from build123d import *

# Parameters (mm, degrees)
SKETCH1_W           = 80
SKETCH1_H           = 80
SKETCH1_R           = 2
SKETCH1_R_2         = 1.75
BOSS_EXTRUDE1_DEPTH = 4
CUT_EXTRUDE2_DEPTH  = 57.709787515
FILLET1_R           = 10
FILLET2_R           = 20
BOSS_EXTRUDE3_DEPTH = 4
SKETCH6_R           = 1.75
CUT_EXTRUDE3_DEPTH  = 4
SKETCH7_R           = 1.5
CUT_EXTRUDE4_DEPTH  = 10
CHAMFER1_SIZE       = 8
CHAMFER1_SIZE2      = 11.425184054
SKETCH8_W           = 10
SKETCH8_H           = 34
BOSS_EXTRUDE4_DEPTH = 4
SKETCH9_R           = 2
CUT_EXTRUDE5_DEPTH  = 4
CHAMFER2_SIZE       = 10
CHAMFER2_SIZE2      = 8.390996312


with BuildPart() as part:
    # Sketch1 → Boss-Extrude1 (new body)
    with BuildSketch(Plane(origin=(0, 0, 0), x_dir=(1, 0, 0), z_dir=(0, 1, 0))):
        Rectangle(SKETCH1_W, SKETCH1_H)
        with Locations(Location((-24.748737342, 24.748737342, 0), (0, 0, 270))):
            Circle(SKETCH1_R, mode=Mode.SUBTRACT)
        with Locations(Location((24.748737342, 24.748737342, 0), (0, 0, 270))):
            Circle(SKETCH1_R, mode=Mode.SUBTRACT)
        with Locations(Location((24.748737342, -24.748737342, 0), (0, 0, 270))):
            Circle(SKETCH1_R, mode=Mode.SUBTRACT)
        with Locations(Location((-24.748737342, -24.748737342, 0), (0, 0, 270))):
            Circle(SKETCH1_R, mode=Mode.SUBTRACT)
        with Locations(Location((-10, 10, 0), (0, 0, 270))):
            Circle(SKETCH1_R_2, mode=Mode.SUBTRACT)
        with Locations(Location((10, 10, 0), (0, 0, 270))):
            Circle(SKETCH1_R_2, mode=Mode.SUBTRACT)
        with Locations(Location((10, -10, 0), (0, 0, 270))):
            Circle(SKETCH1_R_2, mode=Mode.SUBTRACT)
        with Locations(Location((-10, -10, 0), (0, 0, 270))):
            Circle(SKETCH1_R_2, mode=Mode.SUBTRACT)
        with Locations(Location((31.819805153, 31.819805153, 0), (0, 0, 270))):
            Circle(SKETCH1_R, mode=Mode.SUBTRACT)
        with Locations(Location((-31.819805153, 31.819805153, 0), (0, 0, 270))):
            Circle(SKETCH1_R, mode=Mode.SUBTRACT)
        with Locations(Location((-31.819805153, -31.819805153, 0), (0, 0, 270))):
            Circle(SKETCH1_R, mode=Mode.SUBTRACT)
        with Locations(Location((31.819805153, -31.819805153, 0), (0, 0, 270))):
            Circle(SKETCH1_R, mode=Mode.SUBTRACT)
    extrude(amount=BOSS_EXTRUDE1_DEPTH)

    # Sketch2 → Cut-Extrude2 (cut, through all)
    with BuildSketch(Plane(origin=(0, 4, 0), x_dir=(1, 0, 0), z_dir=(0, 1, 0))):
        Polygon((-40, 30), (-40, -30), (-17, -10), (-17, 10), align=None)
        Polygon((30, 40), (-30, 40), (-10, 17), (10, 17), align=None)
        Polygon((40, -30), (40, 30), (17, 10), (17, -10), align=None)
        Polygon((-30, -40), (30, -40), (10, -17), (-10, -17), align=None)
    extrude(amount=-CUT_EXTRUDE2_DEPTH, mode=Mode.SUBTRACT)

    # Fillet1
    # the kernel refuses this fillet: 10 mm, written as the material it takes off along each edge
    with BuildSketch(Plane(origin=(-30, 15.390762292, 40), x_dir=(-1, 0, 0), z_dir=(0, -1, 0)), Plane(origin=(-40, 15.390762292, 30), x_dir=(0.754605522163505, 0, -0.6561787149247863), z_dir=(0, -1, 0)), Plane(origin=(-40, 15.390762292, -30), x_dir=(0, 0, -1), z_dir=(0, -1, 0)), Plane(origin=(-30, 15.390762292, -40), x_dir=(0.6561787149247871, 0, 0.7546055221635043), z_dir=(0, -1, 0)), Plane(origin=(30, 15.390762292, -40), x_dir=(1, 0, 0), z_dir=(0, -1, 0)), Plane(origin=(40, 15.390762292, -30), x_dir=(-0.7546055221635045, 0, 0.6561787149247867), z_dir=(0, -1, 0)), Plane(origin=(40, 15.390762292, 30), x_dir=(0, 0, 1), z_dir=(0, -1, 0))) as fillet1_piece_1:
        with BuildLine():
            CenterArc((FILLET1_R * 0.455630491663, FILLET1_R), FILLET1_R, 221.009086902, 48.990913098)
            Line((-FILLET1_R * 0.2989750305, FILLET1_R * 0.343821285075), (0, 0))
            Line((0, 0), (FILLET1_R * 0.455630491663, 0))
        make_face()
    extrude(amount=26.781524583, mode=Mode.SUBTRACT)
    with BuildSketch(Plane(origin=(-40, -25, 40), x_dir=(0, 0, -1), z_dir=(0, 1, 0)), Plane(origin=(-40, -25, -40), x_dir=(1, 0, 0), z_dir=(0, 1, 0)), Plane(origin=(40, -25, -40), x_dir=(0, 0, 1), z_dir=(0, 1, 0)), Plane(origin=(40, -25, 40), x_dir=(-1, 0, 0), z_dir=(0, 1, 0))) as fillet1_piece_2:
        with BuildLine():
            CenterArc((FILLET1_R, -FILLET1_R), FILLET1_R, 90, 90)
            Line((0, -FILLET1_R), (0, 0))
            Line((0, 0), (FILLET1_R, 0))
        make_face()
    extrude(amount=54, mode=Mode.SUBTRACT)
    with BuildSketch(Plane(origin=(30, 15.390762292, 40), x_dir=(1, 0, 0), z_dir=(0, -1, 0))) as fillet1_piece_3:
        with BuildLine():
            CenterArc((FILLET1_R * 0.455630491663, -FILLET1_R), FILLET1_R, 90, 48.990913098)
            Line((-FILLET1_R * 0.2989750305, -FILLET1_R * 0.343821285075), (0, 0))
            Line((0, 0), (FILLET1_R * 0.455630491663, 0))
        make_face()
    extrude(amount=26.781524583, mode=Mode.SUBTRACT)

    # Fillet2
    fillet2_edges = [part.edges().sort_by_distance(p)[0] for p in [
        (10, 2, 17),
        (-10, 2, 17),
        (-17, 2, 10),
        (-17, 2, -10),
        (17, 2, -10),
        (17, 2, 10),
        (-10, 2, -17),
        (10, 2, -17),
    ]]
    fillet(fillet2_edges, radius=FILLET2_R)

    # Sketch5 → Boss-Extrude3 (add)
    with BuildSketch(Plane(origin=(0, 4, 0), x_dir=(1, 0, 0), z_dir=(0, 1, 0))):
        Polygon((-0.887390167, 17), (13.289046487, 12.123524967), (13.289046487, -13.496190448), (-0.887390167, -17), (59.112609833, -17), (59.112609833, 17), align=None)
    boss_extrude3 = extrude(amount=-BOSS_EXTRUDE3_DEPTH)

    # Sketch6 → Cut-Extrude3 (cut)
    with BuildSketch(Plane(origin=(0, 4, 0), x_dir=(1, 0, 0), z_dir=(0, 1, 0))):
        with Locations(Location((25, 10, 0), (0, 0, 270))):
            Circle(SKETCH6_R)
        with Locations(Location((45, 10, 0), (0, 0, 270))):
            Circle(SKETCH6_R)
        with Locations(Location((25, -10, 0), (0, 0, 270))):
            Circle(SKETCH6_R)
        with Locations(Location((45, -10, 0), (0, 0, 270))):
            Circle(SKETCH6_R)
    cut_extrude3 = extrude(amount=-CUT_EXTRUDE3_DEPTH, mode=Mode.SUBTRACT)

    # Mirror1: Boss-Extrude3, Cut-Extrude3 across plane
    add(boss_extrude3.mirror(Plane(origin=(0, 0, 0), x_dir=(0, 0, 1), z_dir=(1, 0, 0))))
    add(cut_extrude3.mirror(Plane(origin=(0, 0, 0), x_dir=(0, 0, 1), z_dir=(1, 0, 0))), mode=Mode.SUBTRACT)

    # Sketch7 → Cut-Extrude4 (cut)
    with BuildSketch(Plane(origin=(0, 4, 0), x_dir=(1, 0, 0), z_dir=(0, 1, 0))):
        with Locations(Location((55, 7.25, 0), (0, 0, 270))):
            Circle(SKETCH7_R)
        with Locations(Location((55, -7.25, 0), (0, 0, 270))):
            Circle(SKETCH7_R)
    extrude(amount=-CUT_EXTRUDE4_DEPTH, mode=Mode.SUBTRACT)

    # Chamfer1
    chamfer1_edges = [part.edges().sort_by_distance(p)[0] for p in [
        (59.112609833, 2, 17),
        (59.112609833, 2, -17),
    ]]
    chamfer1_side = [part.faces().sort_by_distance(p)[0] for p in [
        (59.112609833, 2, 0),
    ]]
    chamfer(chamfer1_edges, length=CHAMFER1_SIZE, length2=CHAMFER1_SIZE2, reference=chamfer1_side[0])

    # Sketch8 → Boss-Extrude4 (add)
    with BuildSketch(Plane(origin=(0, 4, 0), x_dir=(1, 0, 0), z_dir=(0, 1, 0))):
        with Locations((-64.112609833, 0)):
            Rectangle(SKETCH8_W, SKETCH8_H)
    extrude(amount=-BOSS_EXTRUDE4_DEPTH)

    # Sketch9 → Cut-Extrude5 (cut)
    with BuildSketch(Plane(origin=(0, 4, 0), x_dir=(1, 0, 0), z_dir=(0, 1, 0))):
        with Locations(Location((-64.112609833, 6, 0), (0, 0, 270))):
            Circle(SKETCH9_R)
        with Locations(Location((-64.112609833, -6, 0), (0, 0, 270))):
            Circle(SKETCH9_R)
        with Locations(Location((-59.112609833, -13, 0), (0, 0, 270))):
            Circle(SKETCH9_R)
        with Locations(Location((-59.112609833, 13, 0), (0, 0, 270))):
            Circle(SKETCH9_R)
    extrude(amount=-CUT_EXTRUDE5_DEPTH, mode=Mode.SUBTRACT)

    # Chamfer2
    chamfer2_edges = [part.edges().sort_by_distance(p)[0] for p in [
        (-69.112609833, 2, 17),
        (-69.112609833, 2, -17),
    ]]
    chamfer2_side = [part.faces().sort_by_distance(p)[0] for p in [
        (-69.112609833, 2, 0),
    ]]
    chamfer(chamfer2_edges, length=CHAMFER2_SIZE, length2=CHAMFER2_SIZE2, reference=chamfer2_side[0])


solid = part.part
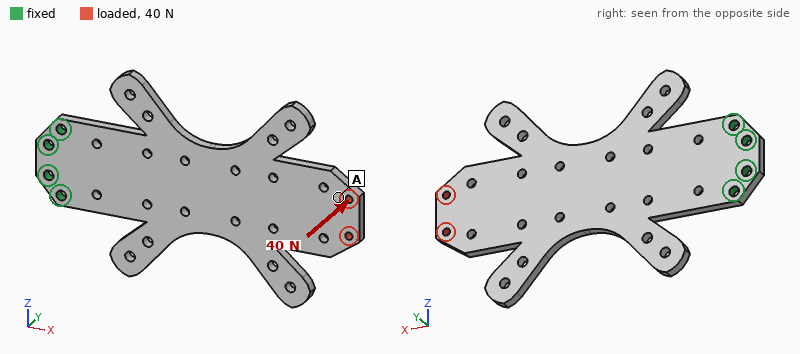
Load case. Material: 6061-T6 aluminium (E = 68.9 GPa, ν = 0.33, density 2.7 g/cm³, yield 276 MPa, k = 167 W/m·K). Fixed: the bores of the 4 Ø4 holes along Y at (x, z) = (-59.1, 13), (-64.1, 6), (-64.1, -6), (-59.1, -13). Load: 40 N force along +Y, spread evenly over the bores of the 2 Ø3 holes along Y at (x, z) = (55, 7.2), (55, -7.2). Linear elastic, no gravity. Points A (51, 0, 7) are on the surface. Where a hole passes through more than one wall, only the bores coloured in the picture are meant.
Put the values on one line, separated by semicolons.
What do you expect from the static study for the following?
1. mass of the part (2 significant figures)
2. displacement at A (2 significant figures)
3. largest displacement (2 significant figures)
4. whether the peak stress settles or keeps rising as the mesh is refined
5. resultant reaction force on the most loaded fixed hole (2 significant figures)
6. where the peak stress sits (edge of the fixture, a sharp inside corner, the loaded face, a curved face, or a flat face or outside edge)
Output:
57 g; 1.5 mm; 1.7 mm; keeps rising; 86 N; edge of the fixture
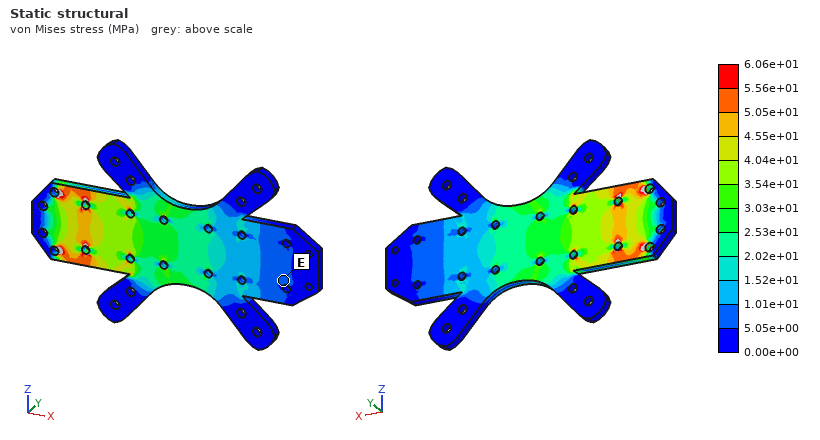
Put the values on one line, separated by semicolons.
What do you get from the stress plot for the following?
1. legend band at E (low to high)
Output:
5.05e+00 to 1.01e+01 MPa
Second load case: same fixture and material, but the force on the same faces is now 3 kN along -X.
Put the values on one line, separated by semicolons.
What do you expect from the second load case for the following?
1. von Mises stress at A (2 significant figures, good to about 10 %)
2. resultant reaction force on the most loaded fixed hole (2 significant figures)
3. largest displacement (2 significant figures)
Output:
38 MPa; 950 N; 43 µm
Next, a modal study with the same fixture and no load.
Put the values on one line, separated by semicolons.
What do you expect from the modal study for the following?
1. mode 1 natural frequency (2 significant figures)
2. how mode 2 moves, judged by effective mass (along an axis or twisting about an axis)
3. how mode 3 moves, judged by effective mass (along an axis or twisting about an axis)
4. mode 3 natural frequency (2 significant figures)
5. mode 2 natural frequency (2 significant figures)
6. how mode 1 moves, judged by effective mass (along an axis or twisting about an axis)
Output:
220 Hz; twisting about X; along Y; 1400 Hz; 850 Hz; along Y
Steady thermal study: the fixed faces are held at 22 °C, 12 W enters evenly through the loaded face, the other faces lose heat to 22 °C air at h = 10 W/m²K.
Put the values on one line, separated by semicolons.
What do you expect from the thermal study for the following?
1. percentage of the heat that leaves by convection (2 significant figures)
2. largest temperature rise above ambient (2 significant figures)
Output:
26 %; 54 K
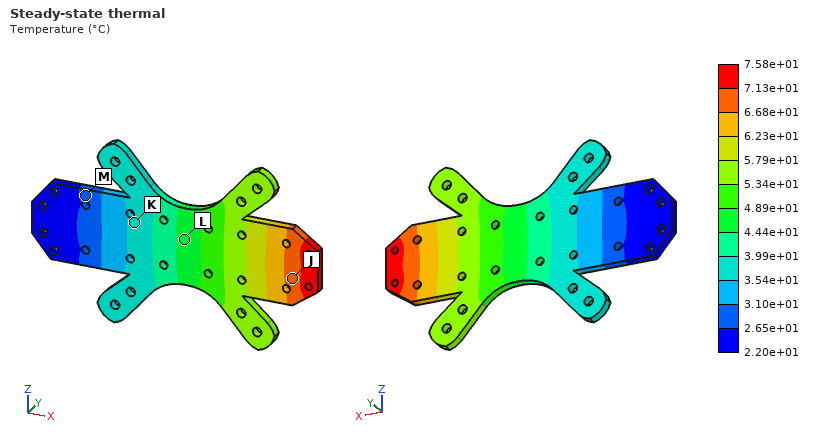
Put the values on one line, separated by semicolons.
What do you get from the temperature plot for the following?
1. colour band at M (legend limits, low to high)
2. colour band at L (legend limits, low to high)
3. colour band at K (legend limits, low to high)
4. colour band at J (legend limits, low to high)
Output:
2.65e+01 to 3.10e+01 °C; 4.44e+01 to 4.89e+01 °C; 3.54e+01 to 3.99e+01 °C; 6.68e+01 to 7.13e+01 °C
